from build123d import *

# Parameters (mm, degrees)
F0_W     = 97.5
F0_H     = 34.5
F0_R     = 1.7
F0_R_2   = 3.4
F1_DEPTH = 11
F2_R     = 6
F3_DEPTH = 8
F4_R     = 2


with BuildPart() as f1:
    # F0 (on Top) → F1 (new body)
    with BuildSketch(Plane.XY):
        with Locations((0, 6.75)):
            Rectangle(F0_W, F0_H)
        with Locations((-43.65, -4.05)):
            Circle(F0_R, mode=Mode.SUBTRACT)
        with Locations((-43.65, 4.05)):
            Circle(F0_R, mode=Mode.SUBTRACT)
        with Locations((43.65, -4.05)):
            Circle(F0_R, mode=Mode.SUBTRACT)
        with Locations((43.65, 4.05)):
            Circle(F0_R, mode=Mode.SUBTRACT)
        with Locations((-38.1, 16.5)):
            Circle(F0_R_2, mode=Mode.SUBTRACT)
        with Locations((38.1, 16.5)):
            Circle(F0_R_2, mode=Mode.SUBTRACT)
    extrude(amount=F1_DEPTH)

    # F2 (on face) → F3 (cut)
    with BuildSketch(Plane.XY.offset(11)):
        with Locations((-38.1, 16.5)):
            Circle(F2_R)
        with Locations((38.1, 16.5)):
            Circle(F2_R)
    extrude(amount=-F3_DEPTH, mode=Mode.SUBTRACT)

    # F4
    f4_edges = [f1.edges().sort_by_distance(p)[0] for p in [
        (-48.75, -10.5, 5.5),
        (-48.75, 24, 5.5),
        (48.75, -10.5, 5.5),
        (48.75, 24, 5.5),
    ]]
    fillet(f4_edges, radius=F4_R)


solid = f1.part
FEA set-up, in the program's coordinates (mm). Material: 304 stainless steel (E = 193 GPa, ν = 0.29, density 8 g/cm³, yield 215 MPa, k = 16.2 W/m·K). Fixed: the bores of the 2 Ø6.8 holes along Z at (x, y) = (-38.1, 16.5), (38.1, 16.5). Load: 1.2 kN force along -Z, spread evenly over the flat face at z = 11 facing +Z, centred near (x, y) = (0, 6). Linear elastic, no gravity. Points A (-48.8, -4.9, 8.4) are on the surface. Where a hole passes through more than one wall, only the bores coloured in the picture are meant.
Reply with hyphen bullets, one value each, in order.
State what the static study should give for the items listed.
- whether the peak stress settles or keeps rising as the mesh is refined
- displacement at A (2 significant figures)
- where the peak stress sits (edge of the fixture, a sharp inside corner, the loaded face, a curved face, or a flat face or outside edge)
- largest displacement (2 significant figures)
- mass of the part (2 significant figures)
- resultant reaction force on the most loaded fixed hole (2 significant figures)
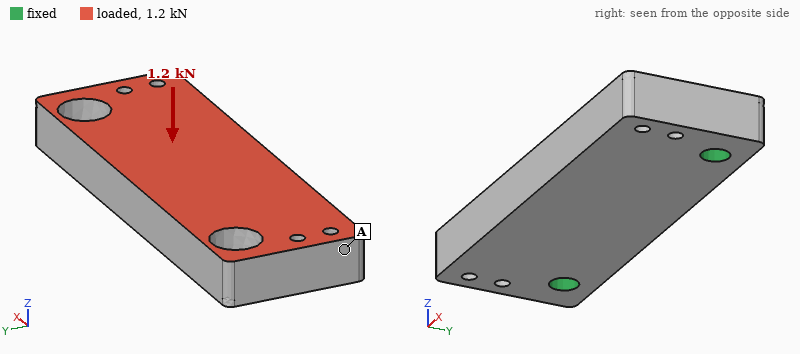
- keeps rising
- 10 µm
- edge of the fixture
- 20 µm
- 280 g
- 730 N
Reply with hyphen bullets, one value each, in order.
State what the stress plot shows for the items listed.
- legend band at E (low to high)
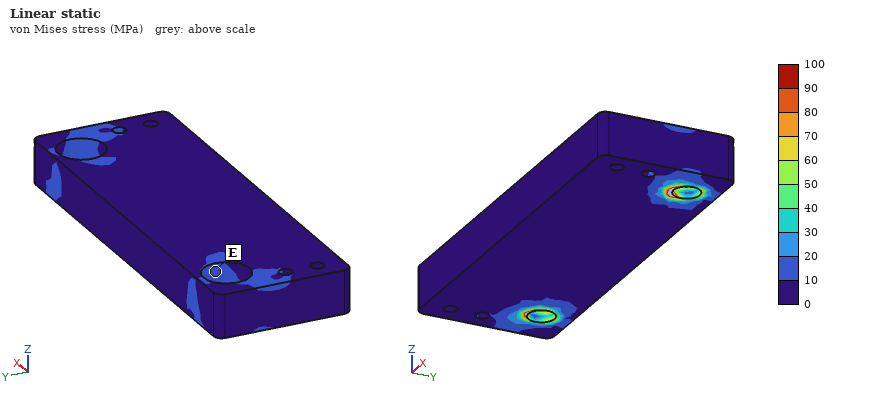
- 10 to 20 MPa
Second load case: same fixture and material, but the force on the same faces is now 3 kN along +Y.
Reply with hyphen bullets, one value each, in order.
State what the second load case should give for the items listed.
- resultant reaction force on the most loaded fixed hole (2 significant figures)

- 1.6 kN
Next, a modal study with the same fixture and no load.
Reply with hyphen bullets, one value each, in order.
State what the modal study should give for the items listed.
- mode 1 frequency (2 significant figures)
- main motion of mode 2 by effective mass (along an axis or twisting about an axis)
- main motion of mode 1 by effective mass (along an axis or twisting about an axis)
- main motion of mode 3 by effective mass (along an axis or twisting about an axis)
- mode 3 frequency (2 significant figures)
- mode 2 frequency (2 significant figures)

- 2900 Hz
- along Z
- along Z
- twisting about Y
- 7100 Hz
- 6600 Hz
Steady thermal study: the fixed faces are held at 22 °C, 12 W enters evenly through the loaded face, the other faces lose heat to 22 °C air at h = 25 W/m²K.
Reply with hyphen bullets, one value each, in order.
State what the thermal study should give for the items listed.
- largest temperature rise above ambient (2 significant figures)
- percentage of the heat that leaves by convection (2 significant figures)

- 28 K
- 29 %
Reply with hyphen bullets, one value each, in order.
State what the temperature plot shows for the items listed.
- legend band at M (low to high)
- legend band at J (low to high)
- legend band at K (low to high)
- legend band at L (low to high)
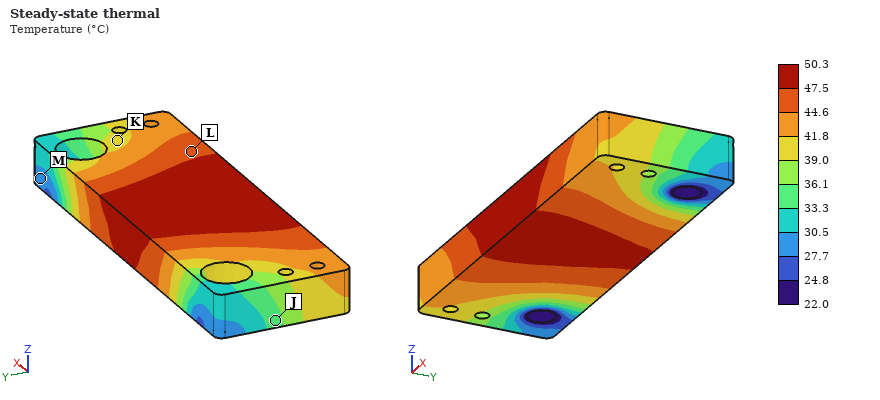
- 27.7 to 30.5 °C
- 33.3 to 36.1 °C
- 39.0 to 41.8 °C
- 44.6 to 47.5 °C
